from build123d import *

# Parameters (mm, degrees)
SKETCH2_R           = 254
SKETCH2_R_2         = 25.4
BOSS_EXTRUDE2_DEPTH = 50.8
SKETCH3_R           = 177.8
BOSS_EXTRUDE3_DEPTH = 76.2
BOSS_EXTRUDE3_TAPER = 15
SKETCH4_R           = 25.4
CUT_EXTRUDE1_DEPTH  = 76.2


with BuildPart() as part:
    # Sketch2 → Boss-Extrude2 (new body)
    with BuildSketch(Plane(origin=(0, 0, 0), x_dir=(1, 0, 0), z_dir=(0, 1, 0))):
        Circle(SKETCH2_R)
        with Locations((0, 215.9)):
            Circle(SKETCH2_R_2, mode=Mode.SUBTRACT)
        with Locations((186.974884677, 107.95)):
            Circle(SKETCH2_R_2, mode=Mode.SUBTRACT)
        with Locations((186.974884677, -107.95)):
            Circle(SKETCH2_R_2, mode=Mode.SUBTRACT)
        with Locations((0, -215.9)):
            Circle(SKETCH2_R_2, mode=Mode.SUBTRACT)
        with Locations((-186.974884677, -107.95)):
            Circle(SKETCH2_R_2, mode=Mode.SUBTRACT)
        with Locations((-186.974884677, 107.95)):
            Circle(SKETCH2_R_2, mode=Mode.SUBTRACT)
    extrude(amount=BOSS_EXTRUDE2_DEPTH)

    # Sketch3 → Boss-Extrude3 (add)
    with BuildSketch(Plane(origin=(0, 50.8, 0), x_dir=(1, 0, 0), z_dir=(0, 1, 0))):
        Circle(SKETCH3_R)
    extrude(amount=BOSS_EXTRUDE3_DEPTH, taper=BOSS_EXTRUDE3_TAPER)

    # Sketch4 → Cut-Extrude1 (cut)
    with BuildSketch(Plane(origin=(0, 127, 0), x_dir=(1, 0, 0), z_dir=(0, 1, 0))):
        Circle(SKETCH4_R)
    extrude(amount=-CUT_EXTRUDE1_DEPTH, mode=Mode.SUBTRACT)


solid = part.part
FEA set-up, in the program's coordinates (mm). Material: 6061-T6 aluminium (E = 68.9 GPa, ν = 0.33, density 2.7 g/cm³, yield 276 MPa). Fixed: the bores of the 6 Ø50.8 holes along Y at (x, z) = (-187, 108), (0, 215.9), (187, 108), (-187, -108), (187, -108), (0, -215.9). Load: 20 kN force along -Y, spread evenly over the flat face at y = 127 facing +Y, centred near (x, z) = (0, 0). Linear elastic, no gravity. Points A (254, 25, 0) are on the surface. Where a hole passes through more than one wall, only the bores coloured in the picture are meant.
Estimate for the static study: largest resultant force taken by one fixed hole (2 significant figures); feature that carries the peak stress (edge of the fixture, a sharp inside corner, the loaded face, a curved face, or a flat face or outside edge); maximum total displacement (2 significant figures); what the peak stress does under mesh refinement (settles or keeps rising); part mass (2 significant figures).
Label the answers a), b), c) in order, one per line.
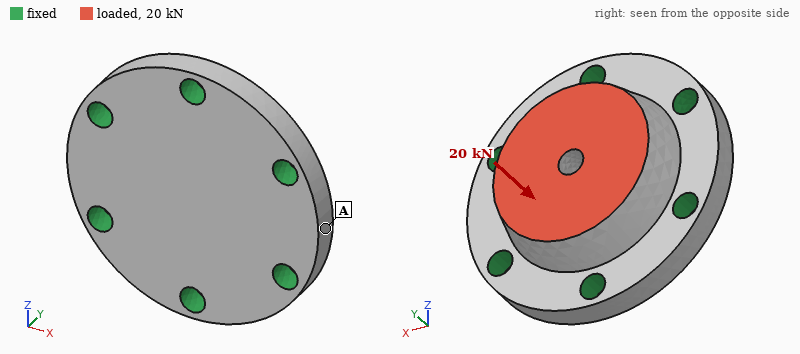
a) 3.8 kN
b) edge of the fixture
c) 2.7 µm
d) keeps rising
e) 44 kg
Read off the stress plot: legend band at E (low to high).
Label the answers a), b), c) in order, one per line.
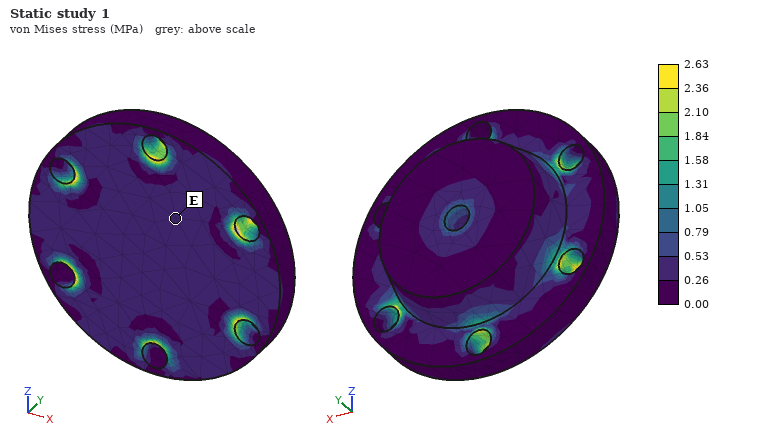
a) 0.26 to 0.53 MPa
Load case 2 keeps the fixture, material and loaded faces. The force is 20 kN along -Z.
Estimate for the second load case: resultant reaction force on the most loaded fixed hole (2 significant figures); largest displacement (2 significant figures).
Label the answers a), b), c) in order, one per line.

a) 5.9 kN
b) 2.5 µm
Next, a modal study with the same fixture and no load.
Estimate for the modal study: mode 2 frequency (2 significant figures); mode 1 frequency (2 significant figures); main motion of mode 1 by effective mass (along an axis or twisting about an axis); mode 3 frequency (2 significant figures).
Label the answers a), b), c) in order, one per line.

a) 3900 Hz
b) 2800 Hz
c) along Y
d) 3900 Hz
